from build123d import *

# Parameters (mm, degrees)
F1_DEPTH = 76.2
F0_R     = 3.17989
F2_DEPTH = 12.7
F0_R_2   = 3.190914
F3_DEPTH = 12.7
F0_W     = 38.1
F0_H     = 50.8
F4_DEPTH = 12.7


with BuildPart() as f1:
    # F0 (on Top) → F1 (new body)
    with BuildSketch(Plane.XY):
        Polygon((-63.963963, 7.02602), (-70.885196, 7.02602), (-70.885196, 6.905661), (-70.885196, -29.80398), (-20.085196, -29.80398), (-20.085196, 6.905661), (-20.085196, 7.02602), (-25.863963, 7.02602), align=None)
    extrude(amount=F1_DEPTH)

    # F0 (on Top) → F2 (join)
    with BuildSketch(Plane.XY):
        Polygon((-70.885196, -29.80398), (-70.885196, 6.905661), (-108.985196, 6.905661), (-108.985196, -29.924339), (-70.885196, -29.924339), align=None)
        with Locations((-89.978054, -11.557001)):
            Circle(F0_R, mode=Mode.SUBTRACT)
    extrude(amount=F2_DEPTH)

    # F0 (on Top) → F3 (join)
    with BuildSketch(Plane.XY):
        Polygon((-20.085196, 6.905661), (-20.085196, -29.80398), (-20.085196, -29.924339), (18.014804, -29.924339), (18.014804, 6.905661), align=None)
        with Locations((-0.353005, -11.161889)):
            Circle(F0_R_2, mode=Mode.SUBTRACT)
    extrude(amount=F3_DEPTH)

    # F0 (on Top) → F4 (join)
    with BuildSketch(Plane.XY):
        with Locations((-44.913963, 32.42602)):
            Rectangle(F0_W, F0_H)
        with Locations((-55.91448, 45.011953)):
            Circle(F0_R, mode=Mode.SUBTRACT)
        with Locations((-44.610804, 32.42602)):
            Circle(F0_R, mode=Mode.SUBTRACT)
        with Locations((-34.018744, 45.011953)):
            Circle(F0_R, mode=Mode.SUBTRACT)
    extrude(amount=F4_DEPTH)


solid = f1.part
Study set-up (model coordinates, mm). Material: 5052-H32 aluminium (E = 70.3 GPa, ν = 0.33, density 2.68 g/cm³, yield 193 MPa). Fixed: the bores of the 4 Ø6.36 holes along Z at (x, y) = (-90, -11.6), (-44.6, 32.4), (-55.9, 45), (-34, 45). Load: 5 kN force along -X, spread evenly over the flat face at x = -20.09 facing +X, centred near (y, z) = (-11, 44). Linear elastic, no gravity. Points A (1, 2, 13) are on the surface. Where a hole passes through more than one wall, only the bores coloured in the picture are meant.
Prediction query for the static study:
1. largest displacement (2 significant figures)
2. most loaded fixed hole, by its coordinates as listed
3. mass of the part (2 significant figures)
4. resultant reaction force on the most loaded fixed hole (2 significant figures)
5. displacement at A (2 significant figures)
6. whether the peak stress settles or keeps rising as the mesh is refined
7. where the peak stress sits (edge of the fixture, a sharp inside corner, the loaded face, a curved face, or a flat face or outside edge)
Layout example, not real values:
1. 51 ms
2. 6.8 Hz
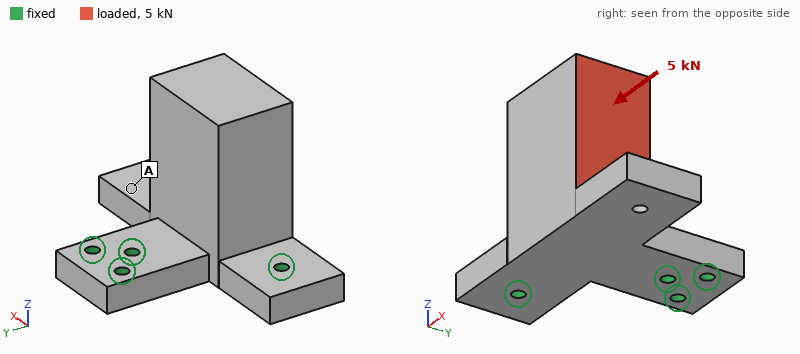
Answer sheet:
1. 0.31 mm
2. (-90, -11.6)
3. 540 g
4. 5.1 kN
5. 0.19 mm
6. keeps rising
7. edge of the fixture
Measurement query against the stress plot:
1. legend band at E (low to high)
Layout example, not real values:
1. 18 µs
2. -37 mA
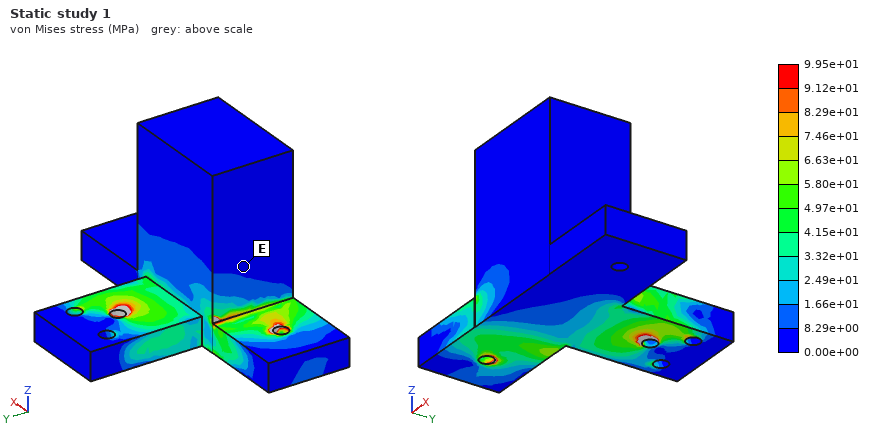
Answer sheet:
1. 0.00e+00 to 8.29e+00 MPa
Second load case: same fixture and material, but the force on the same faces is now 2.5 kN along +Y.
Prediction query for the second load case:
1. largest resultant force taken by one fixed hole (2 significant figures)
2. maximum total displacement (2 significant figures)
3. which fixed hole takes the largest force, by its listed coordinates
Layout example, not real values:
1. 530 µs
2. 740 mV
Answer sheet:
1. 1.9 kN
2. 0.18 mm
3. (-44.6, 32.4)
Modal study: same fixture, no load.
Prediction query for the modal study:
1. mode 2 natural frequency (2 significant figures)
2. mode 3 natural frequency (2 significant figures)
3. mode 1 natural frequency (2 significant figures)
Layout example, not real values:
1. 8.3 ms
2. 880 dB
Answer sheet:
1. 2300 Hz
2. 4400 Hz
3. 990 Hz
